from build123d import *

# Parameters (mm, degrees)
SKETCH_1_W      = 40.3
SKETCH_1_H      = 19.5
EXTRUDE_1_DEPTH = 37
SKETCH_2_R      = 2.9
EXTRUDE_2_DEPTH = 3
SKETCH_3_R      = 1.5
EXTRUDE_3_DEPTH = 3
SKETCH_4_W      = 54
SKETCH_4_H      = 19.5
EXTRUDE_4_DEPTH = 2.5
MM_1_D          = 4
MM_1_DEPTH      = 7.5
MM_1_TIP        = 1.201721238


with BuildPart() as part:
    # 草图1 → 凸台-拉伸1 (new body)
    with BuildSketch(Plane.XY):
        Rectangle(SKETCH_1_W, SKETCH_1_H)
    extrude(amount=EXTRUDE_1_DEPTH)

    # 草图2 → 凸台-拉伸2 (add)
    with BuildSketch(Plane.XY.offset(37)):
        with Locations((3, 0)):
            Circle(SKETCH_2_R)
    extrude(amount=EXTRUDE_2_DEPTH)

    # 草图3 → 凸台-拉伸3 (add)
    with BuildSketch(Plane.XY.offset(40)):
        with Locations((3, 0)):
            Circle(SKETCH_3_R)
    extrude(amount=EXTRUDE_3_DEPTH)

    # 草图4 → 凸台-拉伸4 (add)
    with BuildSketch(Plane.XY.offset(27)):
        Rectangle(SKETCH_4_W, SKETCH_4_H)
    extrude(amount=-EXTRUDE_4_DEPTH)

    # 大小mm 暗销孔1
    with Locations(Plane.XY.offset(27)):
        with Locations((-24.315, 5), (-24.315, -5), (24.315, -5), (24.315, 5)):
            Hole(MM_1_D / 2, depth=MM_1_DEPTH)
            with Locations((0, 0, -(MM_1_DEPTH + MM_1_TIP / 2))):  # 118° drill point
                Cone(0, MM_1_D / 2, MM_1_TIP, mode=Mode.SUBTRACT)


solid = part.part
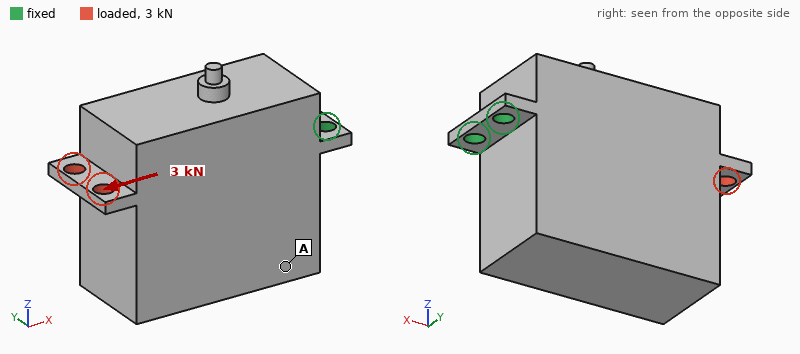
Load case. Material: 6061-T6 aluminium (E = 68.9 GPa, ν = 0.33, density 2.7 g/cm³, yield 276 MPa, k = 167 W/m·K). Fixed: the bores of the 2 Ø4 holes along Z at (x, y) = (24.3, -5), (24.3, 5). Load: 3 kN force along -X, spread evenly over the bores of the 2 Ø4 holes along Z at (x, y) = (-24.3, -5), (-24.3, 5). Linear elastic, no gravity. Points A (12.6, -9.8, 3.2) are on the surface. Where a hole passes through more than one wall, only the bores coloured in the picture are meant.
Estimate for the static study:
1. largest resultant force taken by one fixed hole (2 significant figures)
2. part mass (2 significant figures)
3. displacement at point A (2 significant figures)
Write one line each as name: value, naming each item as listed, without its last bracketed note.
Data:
largest resultant force taken by one fixed hole: 1.5 kN
part mass: 80 g
displacement at point A: 7.3 µm
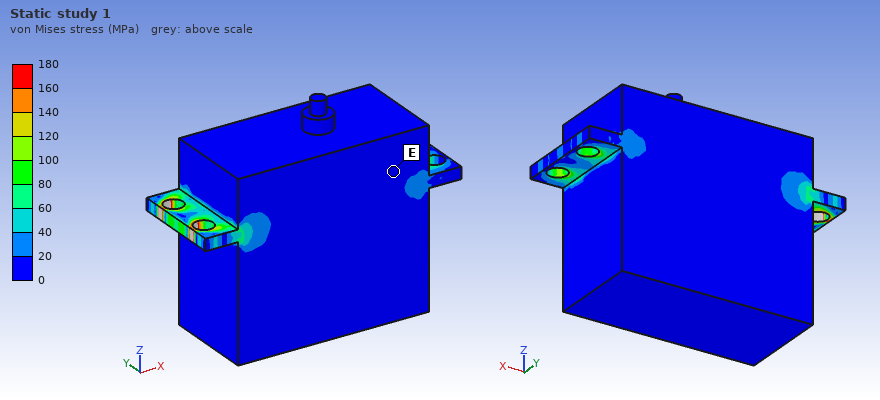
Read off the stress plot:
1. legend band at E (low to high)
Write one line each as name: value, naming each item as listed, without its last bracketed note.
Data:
legend band at E: 0 to 20 MPa
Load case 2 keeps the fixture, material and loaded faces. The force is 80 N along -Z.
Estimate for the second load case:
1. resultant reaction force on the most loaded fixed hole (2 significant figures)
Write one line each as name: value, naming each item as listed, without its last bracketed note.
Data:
resultant reaction force on the most loaded fixed hole: 40 N
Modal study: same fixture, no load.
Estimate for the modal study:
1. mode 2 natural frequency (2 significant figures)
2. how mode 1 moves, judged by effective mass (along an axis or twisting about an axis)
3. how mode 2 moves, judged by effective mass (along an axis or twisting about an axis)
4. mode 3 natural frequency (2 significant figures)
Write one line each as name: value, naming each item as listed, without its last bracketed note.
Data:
mode 2 natural frequency: 2200 Hz
how mode 1 moves, judged by effective mass: along Z
how mode 2 moves, judged by effective mass: along Y
mode 3 natural frequency: 3500 Hz
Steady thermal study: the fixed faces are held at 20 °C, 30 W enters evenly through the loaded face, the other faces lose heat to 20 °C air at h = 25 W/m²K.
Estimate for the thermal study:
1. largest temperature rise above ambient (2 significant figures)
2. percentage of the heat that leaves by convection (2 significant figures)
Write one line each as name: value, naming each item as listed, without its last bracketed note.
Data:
largest temperature rise above ambient: 60 K
percentage of the heat that leaves by convection: 12 %
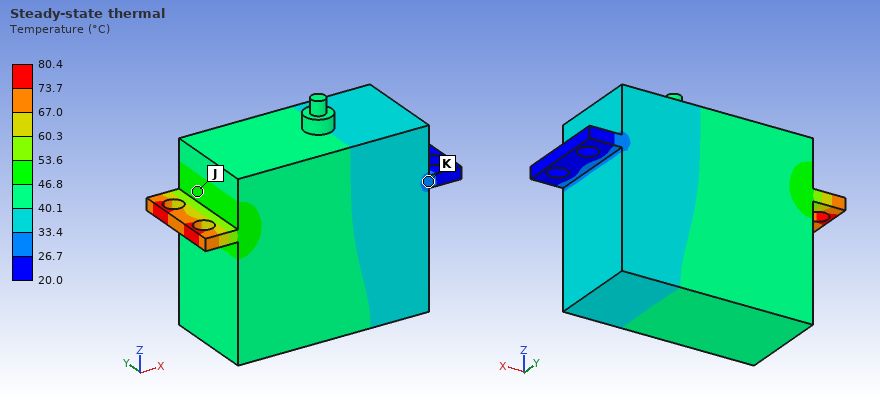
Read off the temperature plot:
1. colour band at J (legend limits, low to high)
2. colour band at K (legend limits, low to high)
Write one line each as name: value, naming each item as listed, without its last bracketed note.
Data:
colour band at J: 46.8 to 53.6 °C
colour band at K: 26.7 to 33.4 °C
